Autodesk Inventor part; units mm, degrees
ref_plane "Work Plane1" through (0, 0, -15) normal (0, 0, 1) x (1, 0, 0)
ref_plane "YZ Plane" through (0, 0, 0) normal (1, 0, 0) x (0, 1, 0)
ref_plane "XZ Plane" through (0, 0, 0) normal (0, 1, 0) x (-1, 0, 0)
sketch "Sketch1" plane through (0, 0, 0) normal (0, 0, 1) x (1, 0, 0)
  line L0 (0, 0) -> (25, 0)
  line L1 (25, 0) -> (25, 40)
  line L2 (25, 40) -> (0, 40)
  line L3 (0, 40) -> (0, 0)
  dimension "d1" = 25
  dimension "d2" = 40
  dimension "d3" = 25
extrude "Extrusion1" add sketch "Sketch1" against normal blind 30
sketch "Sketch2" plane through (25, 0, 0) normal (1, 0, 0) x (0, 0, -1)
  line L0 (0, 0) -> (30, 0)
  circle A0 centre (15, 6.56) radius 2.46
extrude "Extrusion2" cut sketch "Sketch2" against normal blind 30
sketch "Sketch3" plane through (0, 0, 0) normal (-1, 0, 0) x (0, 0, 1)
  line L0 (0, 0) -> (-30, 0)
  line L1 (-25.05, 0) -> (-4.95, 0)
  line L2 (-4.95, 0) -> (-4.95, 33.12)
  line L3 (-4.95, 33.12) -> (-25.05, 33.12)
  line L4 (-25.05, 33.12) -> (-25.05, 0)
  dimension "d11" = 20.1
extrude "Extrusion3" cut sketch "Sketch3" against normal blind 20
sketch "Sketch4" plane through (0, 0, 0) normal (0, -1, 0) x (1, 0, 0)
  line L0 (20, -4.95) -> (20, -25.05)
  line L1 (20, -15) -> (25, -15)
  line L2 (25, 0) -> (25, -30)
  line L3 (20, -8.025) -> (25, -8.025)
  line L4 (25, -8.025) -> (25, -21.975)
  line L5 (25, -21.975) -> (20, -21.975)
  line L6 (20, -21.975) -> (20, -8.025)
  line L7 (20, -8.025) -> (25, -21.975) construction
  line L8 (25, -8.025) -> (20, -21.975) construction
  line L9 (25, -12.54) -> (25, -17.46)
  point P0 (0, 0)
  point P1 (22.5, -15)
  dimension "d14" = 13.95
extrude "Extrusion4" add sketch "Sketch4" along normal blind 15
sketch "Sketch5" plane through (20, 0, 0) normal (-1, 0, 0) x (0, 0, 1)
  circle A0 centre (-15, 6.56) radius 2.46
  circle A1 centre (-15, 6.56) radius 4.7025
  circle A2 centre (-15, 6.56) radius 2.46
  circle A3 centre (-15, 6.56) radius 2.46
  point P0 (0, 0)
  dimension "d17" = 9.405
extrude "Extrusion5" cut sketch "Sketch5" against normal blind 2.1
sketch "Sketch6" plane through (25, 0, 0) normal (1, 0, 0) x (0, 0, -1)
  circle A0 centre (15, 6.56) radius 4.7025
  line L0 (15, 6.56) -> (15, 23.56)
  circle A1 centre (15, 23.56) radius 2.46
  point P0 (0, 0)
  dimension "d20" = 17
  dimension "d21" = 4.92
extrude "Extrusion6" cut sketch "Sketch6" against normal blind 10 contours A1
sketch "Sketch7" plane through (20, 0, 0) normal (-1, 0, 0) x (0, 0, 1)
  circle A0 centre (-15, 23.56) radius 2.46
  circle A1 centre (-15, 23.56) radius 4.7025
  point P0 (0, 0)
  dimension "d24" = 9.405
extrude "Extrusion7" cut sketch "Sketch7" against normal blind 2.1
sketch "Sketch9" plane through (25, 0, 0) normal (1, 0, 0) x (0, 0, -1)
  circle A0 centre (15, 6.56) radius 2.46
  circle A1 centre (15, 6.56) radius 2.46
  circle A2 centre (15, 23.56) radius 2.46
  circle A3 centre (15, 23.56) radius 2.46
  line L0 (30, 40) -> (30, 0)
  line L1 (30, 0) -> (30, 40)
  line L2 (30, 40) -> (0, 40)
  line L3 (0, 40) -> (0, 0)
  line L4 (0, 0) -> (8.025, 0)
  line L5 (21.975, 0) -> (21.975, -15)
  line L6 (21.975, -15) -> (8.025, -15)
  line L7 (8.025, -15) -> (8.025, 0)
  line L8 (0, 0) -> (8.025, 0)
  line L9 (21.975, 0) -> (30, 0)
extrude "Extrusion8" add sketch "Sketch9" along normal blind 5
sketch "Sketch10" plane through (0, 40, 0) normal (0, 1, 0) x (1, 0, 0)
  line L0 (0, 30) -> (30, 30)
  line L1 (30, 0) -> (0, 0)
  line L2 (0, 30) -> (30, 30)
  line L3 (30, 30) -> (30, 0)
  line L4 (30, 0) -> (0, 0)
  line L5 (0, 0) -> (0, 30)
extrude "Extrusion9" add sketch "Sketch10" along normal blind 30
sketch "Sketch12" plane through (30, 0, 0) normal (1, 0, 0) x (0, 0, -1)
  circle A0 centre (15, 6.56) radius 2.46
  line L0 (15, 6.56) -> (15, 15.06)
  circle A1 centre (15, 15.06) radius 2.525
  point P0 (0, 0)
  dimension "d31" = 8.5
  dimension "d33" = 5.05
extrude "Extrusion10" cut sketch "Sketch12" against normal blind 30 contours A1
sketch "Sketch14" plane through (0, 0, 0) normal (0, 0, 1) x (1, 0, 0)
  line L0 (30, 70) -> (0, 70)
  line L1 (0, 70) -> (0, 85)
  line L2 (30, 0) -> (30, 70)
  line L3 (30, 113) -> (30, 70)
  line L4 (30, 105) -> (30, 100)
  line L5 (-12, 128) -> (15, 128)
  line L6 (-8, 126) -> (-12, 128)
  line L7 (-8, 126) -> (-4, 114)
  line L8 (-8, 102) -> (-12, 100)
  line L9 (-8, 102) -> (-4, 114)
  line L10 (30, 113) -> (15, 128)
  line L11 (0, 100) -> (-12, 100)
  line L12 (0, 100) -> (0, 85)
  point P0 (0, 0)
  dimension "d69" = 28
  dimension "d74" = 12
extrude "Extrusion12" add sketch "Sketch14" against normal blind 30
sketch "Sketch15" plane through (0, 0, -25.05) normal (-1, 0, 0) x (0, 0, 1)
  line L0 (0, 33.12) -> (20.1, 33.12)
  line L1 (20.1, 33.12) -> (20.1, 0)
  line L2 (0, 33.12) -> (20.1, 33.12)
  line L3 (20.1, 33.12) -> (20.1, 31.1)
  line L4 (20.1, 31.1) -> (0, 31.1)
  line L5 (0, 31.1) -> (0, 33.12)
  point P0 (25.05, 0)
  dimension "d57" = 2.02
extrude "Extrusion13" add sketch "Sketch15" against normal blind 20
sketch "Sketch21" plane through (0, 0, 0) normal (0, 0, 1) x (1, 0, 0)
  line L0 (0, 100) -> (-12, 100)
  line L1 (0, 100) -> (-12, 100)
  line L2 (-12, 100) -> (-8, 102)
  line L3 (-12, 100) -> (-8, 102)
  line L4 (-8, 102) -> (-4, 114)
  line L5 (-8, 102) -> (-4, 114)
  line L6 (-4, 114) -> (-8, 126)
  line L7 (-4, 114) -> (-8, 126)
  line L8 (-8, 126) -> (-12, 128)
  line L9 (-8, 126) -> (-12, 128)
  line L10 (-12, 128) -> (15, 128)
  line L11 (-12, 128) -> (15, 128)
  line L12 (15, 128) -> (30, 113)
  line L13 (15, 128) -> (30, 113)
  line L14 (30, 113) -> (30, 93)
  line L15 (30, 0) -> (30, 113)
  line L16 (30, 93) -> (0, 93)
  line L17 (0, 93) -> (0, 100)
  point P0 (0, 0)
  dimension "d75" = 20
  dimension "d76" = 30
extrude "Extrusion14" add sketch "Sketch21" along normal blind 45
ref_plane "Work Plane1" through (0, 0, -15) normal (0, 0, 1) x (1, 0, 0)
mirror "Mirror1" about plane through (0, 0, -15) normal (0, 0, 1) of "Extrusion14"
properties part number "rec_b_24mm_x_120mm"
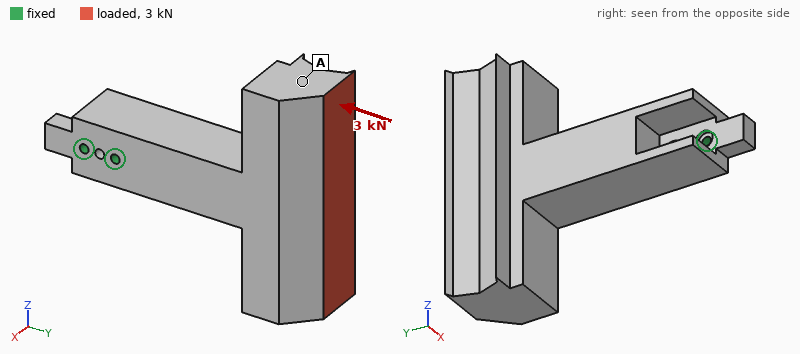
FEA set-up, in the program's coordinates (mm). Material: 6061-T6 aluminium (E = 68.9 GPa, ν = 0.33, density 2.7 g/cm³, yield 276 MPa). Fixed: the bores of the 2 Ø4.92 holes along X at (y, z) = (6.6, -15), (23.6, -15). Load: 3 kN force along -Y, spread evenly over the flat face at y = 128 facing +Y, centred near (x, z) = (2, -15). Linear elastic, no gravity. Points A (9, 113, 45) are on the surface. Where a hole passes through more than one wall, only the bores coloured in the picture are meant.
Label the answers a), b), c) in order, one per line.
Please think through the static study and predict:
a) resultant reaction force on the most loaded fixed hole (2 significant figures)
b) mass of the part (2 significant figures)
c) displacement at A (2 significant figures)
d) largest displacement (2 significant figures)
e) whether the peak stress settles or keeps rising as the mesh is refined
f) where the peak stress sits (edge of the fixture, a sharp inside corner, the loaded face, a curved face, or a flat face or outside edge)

a) 3.4 kN
b) 560 g
c) 0.17 mm
d) 0.22 mm
e) keeps rising
f) edge of the fixture
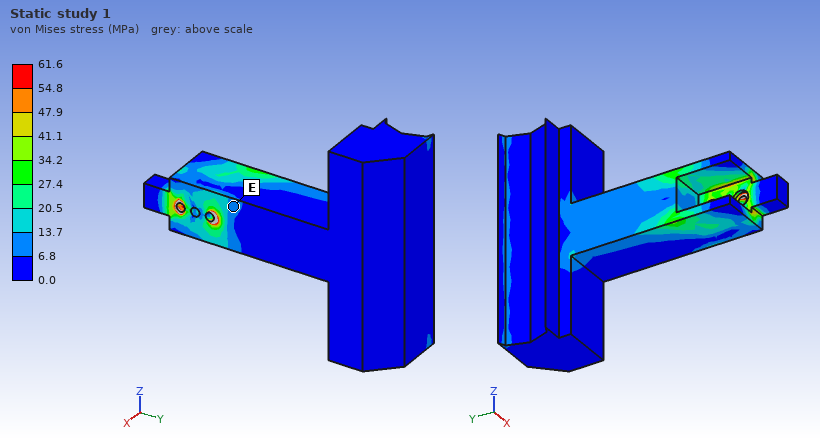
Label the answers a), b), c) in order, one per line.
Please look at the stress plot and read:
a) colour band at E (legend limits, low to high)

a) 6.8 to 13.7 MPa
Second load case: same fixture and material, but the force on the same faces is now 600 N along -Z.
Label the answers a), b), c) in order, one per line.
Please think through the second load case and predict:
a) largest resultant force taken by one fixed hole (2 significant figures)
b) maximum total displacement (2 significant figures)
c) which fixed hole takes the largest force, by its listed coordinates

a) 3.3 kN
b) 0.18 mm
c) (23.6, -15)
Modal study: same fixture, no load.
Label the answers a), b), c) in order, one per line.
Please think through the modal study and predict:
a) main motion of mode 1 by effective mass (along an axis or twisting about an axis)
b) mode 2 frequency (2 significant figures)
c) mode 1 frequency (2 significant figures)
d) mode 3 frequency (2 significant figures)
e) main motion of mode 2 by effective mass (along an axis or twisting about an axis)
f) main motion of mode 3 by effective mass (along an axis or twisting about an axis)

a) along X
b) 590 Hz
c) 540 Hz
d) 860 Hz
e) along Z
f) twisting about Y
